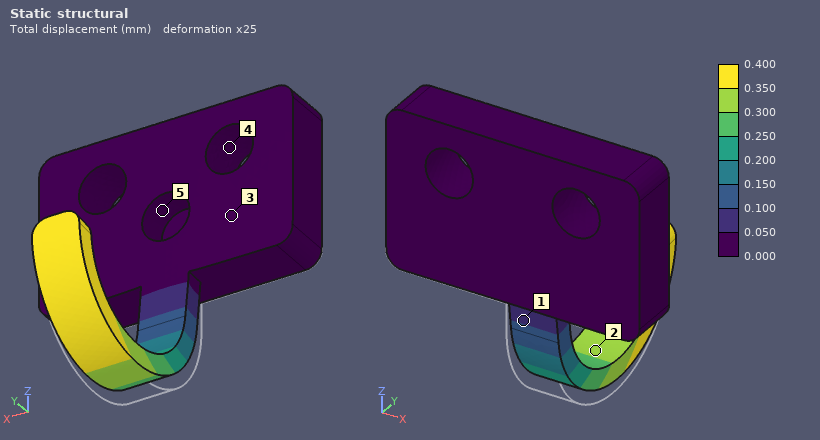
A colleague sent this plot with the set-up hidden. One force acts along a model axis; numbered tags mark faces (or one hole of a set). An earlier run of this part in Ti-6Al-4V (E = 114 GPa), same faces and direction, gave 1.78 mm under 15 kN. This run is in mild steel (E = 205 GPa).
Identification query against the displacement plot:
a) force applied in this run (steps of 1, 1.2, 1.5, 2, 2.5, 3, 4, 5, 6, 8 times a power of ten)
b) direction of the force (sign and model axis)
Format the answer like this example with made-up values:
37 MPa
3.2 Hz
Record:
6 kN
+Y
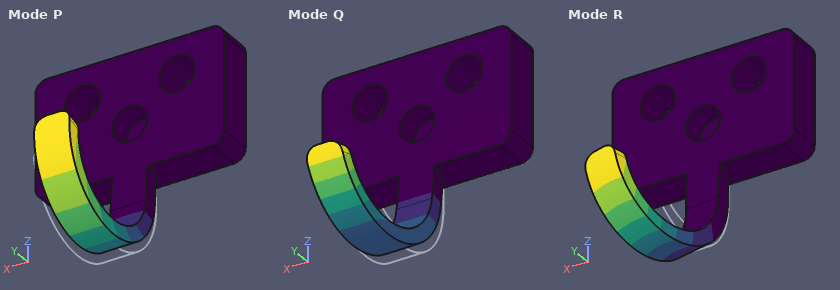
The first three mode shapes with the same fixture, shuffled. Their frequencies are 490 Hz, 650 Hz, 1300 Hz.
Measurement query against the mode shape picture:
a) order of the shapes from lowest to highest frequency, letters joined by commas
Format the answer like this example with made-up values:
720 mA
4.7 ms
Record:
P, R, Q
